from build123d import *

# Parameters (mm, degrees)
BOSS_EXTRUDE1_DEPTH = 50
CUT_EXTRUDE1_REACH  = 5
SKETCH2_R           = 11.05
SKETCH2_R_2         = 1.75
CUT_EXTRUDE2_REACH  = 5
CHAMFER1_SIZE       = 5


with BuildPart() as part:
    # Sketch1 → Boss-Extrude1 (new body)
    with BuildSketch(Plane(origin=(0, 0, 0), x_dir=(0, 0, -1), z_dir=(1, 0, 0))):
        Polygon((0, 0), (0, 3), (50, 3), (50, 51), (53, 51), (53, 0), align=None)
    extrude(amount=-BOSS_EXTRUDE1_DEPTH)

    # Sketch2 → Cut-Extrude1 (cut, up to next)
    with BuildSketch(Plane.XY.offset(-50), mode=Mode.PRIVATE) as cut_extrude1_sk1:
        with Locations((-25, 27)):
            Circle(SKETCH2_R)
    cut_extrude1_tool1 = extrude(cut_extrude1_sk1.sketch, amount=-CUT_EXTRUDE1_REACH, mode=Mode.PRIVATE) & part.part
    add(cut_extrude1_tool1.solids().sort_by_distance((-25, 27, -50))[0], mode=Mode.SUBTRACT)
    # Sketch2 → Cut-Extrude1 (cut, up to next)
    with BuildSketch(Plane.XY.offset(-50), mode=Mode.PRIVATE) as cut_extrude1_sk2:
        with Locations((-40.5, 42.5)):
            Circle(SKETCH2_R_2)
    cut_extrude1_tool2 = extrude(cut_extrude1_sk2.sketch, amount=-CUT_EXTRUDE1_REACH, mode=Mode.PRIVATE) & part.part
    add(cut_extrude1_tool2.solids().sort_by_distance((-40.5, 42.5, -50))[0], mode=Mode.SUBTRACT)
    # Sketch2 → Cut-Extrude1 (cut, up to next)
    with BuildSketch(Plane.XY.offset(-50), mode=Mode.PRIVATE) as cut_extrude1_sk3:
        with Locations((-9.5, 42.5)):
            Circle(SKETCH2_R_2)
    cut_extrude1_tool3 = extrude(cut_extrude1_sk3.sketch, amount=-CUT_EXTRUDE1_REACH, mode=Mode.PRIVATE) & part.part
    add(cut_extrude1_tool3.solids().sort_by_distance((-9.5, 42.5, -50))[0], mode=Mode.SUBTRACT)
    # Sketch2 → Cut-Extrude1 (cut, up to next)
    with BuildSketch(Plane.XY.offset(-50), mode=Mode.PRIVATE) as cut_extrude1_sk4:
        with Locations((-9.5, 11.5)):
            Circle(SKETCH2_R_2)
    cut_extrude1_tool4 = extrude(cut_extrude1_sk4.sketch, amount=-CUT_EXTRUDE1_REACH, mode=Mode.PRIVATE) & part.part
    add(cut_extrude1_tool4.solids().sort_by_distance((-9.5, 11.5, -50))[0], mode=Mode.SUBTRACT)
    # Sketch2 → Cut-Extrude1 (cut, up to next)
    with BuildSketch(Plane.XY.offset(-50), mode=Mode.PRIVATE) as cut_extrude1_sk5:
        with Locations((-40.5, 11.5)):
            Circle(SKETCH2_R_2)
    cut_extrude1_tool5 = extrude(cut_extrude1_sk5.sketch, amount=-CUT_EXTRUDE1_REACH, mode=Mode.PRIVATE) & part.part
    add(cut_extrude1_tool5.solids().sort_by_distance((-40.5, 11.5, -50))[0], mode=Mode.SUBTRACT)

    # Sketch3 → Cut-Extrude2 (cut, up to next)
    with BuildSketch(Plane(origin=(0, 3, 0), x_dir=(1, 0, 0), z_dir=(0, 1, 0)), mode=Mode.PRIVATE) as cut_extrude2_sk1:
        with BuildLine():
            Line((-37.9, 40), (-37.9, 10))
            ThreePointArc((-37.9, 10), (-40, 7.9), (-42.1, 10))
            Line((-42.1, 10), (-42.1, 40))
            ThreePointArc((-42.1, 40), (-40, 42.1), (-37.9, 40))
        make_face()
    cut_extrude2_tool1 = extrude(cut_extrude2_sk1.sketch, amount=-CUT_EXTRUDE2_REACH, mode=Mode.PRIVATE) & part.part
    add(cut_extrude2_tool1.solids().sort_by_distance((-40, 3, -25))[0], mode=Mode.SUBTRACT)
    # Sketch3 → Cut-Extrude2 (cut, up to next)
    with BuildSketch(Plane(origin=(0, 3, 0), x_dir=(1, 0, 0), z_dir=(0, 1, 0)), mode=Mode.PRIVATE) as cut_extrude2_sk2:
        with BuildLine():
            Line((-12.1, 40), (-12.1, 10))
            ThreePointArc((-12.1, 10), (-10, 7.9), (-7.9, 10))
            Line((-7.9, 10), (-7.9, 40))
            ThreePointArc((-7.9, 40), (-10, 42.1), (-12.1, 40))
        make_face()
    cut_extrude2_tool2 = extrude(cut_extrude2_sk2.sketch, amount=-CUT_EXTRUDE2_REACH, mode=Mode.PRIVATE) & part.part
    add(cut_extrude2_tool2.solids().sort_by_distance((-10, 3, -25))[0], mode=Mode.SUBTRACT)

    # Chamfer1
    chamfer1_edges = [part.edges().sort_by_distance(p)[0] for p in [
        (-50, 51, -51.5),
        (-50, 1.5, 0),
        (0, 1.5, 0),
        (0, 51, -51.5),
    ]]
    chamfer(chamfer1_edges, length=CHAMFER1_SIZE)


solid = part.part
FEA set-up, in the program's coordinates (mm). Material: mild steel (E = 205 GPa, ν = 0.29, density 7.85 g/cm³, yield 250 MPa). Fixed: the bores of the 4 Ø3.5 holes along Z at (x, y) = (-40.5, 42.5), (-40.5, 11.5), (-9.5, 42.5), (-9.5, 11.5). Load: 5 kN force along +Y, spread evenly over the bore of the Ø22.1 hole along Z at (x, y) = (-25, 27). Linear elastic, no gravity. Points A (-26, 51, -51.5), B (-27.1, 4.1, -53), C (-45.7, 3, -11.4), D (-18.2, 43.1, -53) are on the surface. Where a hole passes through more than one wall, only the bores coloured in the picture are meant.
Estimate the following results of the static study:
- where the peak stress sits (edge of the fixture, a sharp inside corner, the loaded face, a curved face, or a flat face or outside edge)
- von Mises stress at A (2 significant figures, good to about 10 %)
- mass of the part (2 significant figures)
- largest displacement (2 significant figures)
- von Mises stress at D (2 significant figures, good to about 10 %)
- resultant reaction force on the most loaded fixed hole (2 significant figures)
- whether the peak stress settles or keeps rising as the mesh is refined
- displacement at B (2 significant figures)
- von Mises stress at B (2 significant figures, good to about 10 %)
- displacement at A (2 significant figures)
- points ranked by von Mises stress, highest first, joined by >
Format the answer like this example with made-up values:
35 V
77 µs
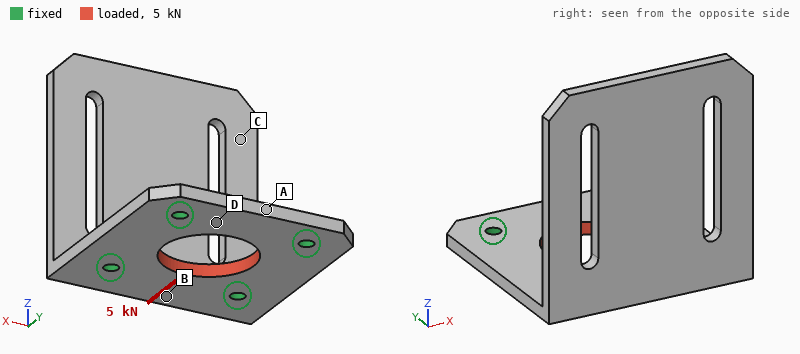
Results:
edge of the fixture
36 MPa
100 g
4.0 µm
25 MPa
1.3 kN
keeps rising
2.3 µm
13 MPa
3.2 µm
A > D > B > C
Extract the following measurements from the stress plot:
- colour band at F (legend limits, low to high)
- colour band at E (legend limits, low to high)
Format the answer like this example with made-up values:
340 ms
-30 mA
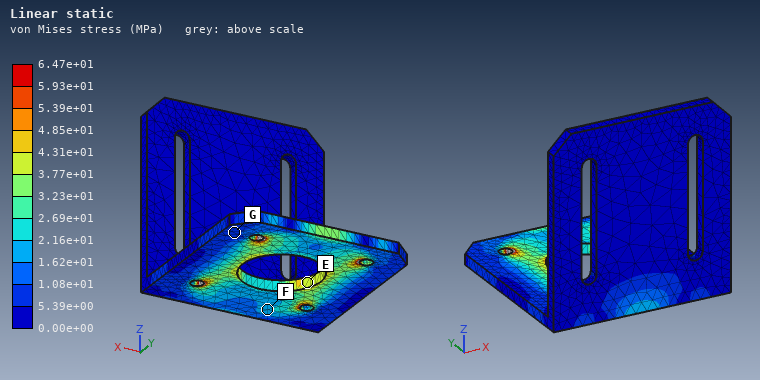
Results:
1.62e+01 to 2.16e+01 MPa
3.77e+01 to 4.31e+01 MPa
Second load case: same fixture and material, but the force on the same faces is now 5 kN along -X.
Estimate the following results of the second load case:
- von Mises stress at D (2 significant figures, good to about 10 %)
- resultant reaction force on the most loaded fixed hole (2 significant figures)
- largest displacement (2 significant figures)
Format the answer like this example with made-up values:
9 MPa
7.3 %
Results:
23 MPa
1.3 kN
3.7 µm
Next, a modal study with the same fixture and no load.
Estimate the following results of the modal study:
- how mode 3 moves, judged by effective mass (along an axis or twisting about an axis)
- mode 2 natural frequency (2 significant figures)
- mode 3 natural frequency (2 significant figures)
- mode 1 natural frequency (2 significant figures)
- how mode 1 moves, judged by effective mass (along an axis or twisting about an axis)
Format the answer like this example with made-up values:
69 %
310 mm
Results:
along X
2000 Hz
3100 Hz
740 Hz
along Y
